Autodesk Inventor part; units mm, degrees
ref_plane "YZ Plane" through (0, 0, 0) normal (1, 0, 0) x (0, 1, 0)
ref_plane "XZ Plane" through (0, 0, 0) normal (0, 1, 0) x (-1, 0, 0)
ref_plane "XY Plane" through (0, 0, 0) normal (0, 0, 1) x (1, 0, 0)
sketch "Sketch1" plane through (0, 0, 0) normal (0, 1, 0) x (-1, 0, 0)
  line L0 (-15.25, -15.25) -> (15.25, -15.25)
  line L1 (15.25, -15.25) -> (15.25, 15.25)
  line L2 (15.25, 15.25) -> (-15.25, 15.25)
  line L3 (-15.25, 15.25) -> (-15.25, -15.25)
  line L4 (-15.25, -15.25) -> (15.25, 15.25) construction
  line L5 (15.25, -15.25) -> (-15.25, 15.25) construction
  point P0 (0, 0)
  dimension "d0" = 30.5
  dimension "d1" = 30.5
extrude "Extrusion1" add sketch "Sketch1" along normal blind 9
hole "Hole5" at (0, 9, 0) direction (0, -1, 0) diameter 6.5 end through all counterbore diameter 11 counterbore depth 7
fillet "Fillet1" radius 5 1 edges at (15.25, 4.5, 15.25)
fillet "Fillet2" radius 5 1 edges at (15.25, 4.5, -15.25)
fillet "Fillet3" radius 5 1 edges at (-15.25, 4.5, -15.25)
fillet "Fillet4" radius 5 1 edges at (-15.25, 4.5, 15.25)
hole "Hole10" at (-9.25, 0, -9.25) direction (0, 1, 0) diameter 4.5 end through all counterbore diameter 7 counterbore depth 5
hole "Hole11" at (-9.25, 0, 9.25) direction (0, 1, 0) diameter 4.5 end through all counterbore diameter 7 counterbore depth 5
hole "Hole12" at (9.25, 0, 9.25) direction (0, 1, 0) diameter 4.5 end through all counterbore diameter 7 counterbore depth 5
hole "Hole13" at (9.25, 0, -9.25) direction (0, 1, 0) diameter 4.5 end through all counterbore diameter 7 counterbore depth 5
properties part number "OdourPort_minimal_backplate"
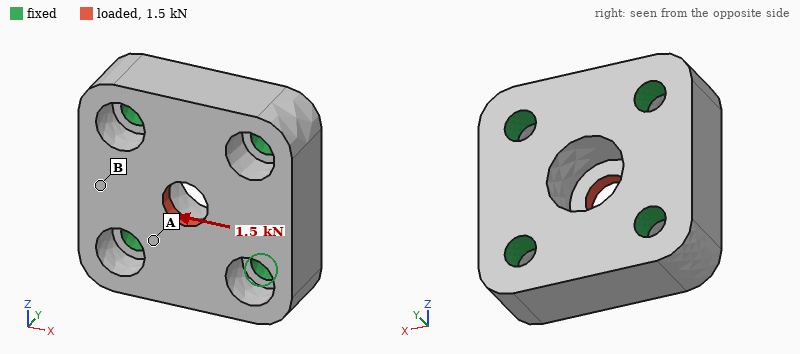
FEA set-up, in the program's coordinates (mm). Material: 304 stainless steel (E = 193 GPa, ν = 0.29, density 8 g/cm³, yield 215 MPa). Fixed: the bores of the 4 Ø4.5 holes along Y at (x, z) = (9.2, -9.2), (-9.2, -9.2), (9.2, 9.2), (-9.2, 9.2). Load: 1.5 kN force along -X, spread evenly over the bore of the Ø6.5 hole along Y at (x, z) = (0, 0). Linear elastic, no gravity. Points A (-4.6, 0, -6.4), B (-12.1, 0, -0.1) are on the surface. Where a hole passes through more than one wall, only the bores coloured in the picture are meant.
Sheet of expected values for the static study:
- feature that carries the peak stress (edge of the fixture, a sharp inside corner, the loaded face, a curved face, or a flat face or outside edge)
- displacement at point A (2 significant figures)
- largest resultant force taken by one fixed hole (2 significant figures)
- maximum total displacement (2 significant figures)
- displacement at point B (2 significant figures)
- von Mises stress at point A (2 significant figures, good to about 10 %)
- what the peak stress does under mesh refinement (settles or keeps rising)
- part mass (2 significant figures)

a sharp inside corner
0.77 µm
430 N
1.9 µm
0.92 µm
14 MPa
keeps rising
51 g
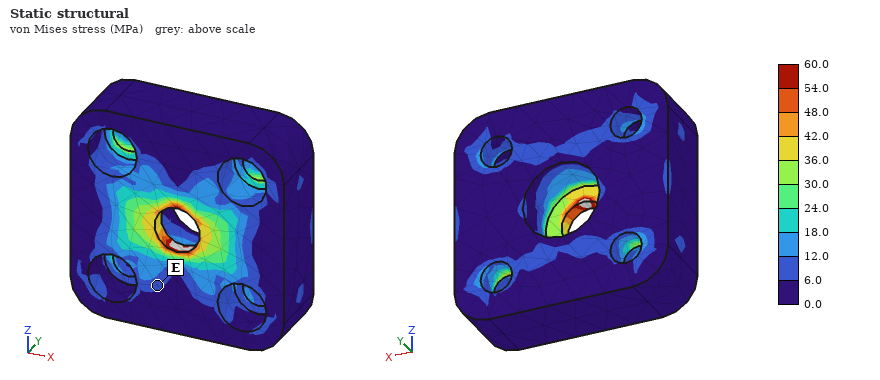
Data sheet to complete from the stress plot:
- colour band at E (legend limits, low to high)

6.0 to 12.0 MPa
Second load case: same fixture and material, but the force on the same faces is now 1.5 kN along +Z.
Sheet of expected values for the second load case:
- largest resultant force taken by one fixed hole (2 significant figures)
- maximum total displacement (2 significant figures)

430 N
1.9 µm
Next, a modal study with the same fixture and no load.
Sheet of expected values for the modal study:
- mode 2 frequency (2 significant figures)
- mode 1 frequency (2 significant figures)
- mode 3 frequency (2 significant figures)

49 kHz
48 kHz
49 kHz
